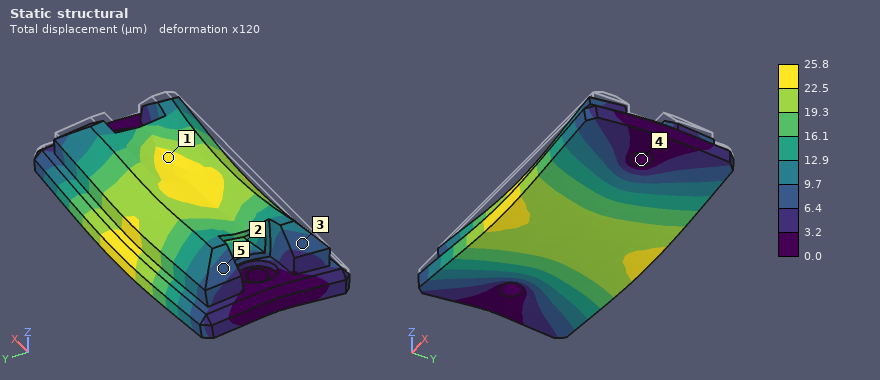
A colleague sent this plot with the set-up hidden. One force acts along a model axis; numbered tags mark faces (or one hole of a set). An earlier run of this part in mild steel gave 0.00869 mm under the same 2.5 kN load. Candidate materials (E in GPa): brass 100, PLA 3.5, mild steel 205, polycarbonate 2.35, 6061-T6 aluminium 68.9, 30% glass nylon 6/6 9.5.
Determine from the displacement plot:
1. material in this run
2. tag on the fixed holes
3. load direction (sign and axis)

6061-T6 aluminium
4
-Z
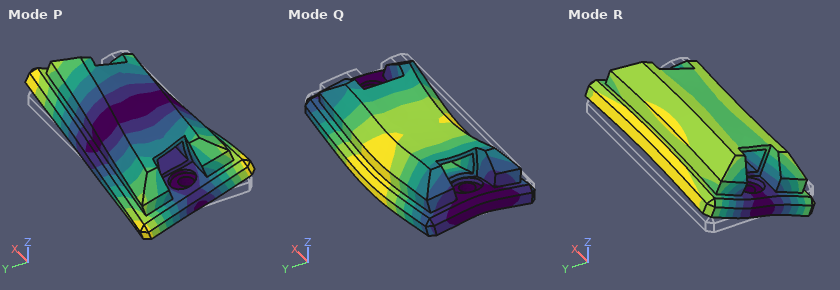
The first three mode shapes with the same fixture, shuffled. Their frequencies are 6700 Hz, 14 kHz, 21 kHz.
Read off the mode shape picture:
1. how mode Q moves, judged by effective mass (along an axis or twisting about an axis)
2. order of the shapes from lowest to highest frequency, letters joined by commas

along Z
R, Q, P
